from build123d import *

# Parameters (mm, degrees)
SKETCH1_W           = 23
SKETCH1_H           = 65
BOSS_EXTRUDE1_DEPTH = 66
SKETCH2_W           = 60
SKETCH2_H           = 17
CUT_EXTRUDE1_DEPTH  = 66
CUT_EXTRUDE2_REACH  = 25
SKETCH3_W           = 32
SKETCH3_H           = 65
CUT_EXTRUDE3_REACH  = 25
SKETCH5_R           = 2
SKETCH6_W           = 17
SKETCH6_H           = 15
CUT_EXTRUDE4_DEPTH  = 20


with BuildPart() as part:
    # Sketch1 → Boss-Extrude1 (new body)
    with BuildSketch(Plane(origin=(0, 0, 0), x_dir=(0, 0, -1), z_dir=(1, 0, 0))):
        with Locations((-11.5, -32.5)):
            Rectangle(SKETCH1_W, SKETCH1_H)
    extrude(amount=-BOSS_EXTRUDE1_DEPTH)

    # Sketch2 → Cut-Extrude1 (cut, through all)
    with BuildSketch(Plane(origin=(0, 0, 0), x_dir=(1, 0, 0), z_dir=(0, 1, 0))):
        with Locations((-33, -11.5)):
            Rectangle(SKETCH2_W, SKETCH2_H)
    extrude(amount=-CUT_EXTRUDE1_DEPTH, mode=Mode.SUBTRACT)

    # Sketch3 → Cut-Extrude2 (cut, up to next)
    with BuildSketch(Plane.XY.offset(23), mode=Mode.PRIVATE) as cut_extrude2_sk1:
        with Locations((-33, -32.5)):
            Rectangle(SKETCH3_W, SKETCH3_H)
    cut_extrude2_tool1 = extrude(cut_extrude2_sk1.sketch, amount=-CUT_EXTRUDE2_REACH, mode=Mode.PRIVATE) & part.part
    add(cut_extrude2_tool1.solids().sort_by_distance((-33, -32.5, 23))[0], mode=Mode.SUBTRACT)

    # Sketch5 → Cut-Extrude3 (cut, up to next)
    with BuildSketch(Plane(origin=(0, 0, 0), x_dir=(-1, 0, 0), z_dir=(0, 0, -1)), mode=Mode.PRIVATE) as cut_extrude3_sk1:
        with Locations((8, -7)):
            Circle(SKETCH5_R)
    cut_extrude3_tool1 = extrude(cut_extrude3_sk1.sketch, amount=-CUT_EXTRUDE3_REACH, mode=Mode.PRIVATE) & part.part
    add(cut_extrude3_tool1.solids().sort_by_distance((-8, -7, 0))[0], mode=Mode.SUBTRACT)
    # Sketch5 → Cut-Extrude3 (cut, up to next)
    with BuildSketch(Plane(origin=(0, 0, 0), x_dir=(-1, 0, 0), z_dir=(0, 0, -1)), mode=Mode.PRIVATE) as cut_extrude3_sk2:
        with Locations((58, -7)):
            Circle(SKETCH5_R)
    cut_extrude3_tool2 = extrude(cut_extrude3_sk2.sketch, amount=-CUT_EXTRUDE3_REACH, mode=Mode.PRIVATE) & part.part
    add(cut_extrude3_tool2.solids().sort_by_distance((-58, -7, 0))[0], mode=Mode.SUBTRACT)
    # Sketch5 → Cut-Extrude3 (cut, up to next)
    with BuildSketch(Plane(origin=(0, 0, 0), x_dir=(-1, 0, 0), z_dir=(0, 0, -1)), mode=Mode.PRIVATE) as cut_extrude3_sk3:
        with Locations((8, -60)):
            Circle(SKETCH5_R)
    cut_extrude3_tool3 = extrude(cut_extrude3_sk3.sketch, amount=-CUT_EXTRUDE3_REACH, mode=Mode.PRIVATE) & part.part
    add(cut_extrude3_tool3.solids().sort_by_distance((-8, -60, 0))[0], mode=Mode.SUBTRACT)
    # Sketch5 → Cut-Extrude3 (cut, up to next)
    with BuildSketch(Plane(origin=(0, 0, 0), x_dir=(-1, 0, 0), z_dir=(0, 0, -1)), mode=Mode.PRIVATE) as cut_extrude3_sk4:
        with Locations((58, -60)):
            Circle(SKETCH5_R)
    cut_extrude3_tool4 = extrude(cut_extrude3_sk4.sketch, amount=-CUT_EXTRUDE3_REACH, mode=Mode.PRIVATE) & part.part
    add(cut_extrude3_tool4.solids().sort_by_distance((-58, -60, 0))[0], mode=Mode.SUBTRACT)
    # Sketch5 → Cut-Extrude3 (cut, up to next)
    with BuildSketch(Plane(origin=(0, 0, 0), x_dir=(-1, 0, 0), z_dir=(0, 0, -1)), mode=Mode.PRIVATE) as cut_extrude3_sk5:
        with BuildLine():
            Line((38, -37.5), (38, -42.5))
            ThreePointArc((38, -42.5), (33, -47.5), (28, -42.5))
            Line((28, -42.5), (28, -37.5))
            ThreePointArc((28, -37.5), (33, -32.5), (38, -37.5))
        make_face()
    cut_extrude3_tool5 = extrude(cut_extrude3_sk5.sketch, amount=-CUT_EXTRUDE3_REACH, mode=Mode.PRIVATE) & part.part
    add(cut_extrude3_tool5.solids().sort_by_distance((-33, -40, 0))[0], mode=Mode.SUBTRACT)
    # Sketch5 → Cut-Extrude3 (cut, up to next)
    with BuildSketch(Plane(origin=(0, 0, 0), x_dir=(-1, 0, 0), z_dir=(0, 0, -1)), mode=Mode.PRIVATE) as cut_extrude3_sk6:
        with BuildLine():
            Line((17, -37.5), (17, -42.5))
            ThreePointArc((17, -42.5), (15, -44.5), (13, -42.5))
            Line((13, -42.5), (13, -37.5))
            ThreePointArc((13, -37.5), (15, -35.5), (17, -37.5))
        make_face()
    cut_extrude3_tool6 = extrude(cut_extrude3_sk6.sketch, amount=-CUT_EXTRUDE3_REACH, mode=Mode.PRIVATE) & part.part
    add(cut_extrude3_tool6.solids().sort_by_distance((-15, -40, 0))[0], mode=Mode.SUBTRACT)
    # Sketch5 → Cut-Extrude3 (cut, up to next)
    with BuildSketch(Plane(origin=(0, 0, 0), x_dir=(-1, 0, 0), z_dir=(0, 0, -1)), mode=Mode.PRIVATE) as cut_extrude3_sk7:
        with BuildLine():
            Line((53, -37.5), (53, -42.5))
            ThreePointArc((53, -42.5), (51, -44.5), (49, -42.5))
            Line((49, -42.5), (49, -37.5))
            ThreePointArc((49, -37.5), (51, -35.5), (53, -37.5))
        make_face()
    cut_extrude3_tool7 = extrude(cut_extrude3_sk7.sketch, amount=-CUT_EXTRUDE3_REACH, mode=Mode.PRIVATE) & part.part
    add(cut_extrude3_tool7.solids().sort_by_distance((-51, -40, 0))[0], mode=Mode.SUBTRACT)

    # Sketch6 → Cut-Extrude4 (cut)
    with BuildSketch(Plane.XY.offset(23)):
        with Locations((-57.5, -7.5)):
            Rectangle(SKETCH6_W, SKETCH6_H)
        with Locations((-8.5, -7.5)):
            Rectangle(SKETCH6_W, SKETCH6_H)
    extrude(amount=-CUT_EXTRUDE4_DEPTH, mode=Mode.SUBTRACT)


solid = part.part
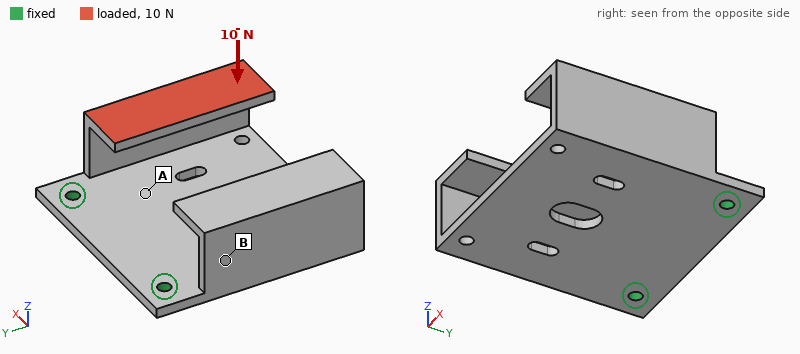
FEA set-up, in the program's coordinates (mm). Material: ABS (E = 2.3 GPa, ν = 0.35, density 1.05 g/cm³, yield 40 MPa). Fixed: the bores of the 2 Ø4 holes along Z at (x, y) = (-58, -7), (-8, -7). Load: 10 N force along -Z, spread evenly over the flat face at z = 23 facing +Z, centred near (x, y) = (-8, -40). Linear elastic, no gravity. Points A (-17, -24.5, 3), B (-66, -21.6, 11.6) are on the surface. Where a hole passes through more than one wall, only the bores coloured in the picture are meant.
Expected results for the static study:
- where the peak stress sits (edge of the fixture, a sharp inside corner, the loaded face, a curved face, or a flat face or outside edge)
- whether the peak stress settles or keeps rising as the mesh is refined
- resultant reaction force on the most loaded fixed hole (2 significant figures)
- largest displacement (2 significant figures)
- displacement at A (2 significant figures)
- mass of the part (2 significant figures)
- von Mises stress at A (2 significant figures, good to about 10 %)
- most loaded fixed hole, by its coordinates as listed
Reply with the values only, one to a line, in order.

edge of the fixture
keeps rising
9.7 N
1.1 mm
0.19 mm
23 g
1.6 MPa
(-8, -7)
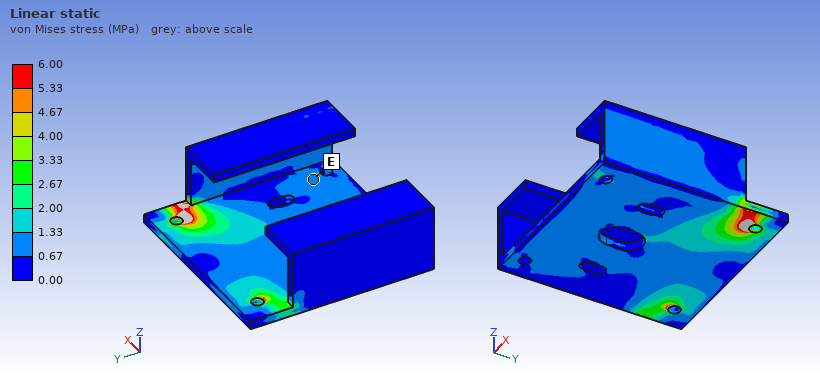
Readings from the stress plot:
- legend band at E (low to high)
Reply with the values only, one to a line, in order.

0.67 to 1.33 MPa
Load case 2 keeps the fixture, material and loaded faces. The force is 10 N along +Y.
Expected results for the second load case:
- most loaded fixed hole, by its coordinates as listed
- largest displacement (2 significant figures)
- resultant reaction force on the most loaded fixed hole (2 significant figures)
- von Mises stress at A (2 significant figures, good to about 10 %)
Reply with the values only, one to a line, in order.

(-8, -7)
1.00 mm
9.8 N
1.6 MPa
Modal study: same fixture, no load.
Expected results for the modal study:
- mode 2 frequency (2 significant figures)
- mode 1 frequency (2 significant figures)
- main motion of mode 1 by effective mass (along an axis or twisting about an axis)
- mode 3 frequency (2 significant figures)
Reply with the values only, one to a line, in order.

240 Hz
150 Hz
along Z
400 Hz
